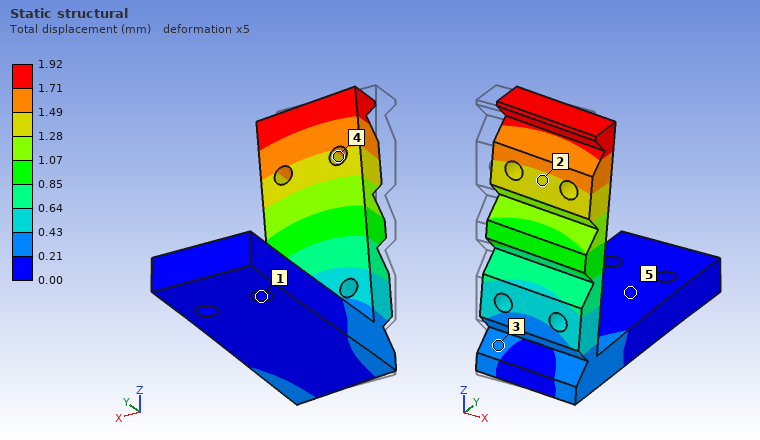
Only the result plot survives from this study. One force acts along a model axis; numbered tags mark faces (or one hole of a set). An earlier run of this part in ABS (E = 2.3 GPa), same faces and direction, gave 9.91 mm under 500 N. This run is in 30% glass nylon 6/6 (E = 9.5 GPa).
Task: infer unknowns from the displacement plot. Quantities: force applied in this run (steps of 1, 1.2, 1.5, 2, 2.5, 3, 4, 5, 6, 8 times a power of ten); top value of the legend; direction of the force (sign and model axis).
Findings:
400 N
1.92 mm
+X
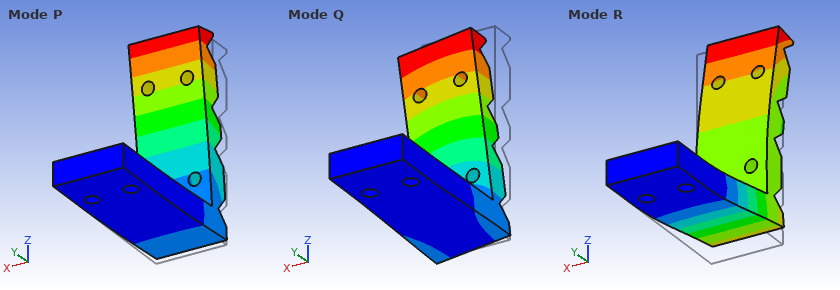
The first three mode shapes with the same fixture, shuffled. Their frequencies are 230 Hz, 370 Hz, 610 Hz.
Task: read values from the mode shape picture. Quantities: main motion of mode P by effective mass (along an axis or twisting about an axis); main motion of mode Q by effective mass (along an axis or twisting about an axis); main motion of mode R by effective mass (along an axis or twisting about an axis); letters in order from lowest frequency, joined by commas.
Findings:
along Y
along X
along Z
P, Q, R
